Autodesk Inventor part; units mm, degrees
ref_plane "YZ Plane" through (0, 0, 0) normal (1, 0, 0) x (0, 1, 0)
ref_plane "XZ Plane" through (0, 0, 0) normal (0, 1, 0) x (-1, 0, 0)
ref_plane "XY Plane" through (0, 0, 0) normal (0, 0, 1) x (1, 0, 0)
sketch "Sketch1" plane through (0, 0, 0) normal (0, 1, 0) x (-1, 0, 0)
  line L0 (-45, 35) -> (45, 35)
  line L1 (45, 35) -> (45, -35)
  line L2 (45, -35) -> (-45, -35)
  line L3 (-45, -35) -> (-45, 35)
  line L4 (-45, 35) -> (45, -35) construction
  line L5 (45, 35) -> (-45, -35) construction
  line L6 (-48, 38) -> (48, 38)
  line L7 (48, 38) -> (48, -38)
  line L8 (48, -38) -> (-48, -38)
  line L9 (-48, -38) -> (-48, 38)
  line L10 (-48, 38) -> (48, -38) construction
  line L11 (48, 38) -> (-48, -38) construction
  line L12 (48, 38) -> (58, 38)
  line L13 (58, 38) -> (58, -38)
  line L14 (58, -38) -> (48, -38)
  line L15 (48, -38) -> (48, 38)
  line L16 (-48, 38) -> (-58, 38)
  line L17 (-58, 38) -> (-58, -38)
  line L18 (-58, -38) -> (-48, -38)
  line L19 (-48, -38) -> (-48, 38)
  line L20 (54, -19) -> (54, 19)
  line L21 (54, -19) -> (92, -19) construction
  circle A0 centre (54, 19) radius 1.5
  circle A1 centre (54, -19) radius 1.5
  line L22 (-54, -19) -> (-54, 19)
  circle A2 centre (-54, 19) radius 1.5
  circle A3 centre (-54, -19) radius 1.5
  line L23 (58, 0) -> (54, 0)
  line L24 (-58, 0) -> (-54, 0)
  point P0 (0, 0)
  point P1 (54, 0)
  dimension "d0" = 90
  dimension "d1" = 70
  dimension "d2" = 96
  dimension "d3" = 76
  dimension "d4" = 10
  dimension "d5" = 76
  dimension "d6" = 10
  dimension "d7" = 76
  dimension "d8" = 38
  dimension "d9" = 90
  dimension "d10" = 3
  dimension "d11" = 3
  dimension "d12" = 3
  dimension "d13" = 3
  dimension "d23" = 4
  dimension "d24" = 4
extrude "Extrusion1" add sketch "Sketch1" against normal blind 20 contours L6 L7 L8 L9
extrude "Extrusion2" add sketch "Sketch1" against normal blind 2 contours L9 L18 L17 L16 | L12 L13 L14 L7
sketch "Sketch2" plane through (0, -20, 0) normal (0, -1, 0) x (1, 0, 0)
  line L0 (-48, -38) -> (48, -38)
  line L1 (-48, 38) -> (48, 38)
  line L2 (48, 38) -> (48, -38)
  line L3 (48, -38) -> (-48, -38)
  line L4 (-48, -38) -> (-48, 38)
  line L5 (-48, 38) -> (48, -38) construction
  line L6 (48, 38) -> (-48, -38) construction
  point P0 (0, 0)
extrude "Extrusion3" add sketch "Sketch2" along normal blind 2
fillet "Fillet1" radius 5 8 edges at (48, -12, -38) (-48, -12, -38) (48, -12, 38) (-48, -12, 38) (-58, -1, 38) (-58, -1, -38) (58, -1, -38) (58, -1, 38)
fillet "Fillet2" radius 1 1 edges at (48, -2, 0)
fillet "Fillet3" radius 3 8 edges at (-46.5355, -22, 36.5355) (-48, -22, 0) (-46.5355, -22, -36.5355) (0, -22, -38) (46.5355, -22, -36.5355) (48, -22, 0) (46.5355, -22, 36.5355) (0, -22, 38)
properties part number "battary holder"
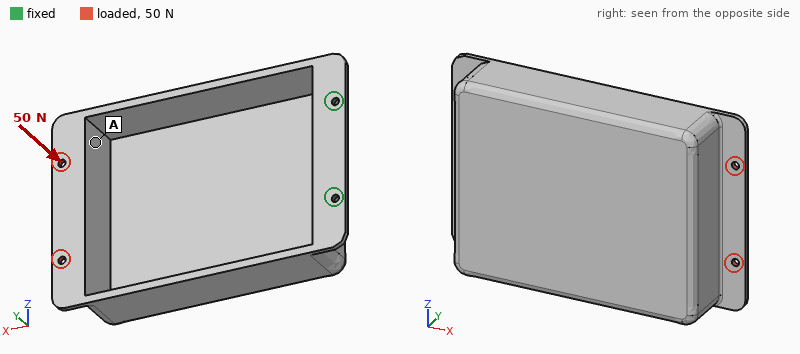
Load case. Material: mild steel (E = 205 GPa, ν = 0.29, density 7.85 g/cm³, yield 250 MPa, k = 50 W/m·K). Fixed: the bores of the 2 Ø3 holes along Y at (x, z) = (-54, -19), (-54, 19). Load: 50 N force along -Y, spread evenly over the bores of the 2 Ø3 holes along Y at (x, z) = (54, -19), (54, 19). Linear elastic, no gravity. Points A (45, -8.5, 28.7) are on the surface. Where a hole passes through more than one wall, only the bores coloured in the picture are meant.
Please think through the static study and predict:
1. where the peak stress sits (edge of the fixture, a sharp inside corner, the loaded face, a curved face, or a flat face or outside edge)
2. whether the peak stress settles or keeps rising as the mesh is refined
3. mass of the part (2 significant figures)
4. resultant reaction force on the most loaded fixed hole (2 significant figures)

edge of the fixture
keeps rising
290 g
190 N
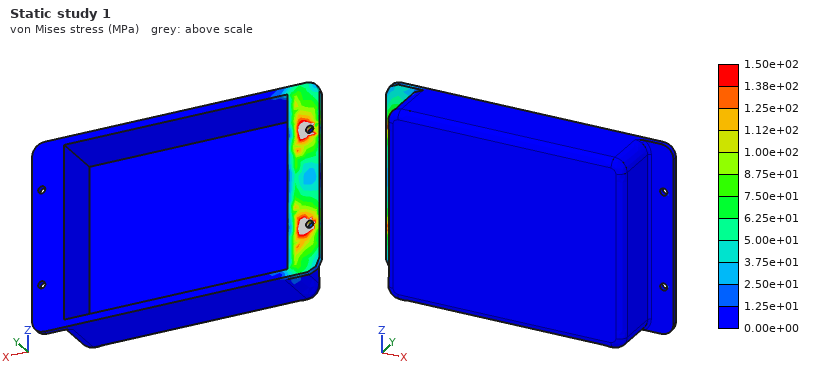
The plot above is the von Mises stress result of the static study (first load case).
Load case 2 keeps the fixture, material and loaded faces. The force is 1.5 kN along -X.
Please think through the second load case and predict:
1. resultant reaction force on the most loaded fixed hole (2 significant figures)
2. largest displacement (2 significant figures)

1.2 kN
0.26 mm
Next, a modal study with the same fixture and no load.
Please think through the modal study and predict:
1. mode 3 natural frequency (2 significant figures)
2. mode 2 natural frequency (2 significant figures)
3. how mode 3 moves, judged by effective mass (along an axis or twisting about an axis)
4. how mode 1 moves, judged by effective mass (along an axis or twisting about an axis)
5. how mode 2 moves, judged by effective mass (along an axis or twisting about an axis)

1300 Hz
360 Hz
along Z
along Y
along Z
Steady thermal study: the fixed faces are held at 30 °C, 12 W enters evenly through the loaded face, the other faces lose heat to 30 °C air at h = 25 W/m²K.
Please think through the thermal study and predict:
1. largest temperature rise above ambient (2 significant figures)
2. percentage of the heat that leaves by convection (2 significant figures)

68 K
92 %
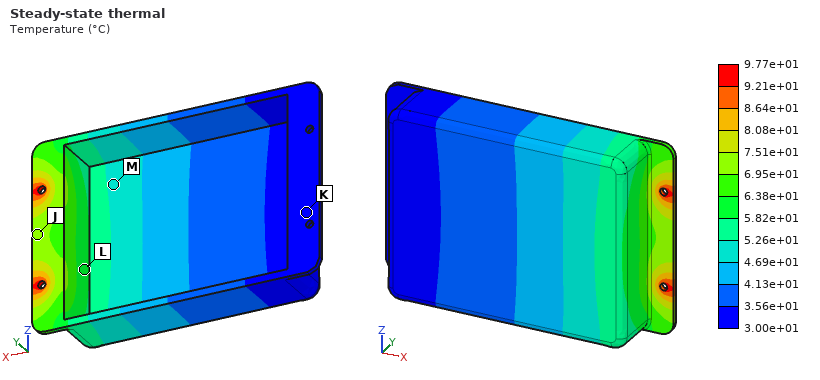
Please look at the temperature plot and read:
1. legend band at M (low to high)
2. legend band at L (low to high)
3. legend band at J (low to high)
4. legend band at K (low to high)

4.69e+01 to 5.26e+01 °C
5.82e+01 to 6.38e+01 °C
6.95e+01 to 7.51e+01 °C
3.00e+01 to 3.56e+01 °C
